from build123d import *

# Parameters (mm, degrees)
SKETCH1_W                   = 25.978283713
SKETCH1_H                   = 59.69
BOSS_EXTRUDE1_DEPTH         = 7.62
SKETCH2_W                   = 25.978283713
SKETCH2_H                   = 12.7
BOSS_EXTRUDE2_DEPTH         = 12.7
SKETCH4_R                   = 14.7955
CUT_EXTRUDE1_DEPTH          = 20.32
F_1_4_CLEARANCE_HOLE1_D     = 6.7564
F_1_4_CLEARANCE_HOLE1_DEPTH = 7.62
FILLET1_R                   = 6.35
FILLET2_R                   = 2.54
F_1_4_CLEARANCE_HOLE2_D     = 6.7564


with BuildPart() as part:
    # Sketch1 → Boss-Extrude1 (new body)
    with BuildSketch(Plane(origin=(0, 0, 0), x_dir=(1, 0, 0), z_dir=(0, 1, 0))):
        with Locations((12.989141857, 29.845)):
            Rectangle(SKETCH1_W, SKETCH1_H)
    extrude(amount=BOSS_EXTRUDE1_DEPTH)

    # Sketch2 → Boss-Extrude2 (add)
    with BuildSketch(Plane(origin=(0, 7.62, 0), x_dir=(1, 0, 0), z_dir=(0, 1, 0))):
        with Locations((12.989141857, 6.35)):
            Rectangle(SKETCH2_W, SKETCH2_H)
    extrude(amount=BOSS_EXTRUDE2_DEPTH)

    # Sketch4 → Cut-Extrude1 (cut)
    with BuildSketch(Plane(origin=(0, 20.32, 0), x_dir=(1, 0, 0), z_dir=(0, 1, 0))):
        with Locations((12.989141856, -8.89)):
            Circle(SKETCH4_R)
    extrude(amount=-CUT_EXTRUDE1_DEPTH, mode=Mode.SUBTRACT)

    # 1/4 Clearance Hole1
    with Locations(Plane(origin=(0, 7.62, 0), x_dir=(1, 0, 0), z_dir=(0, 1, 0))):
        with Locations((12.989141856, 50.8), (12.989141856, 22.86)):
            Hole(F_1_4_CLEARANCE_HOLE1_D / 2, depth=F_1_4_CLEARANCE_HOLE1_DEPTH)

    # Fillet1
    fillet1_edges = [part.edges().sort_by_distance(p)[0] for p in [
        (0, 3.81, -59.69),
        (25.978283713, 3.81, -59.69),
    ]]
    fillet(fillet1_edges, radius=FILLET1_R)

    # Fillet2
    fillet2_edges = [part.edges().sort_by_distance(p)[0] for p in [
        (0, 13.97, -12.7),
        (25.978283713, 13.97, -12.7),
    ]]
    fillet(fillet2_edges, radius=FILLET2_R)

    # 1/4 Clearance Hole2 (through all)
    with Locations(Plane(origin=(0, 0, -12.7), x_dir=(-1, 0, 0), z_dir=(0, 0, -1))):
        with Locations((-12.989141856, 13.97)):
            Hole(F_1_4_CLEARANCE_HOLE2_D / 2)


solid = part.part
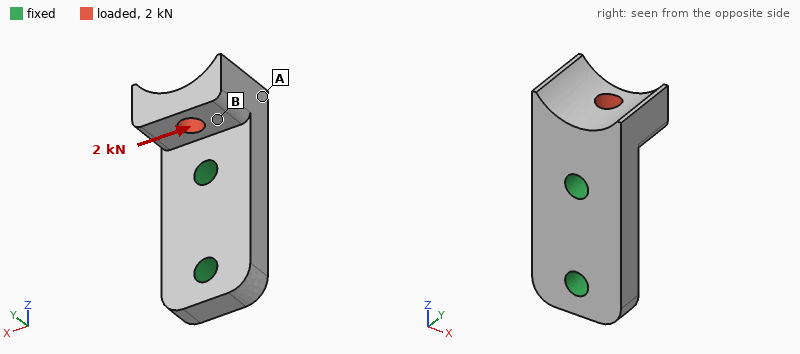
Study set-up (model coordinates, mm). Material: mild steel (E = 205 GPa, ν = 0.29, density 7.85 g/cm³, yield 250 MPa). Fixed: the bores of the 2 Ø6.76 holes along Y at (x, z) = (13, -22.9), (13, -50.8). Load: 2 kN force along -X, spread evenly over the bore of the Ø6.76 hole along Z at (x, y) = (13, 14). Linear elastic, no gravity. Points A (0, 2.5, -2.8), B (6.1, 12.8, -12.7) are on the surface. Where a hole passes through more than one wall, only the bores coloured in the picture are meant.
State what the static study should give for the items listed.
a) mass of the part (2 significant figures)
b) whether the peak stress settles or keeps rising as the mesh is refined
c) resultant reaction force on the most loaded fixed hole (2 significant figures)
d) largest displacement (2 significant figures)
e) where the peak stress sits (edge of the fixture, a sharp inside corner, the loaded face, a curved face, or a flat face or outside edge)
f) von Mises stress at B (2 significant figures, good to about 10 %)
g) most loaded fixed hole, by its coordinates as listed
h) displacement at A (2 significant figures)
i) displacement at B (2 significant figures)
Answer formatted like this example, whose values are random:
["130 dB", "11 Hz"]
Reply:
["100 g", "keeps rising", "2.5 kN", "22 µm", "edge of the fixture", "34 MPa", "(13, -22.9)", "12 µm", "12 µm"]
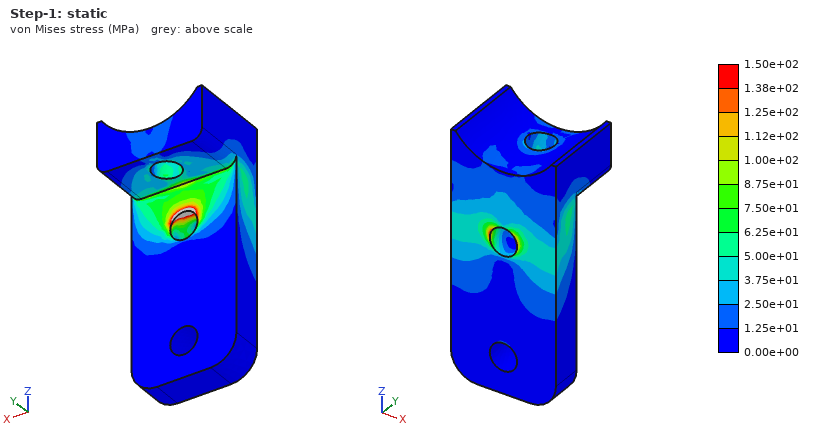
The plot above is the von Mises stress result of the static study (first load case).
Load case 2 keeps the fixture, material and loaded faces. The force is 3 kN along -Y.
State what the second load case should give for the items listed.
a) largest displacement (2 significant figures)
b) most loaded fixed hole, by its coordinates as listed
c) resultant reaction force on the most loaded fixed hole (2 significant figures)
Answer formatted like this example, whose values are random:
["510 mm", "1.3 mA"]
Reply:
["34 µm", "(13, -22.9)", "3.3 kN"]
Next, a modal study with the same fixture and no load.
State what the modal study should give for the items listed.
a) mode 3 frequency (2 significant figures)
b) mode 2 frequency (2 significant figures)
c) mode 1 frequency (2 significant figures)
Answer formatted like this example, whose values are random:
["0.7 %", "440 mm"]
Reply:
["16 kHz", "10 kHz", "8100 Hz"]
